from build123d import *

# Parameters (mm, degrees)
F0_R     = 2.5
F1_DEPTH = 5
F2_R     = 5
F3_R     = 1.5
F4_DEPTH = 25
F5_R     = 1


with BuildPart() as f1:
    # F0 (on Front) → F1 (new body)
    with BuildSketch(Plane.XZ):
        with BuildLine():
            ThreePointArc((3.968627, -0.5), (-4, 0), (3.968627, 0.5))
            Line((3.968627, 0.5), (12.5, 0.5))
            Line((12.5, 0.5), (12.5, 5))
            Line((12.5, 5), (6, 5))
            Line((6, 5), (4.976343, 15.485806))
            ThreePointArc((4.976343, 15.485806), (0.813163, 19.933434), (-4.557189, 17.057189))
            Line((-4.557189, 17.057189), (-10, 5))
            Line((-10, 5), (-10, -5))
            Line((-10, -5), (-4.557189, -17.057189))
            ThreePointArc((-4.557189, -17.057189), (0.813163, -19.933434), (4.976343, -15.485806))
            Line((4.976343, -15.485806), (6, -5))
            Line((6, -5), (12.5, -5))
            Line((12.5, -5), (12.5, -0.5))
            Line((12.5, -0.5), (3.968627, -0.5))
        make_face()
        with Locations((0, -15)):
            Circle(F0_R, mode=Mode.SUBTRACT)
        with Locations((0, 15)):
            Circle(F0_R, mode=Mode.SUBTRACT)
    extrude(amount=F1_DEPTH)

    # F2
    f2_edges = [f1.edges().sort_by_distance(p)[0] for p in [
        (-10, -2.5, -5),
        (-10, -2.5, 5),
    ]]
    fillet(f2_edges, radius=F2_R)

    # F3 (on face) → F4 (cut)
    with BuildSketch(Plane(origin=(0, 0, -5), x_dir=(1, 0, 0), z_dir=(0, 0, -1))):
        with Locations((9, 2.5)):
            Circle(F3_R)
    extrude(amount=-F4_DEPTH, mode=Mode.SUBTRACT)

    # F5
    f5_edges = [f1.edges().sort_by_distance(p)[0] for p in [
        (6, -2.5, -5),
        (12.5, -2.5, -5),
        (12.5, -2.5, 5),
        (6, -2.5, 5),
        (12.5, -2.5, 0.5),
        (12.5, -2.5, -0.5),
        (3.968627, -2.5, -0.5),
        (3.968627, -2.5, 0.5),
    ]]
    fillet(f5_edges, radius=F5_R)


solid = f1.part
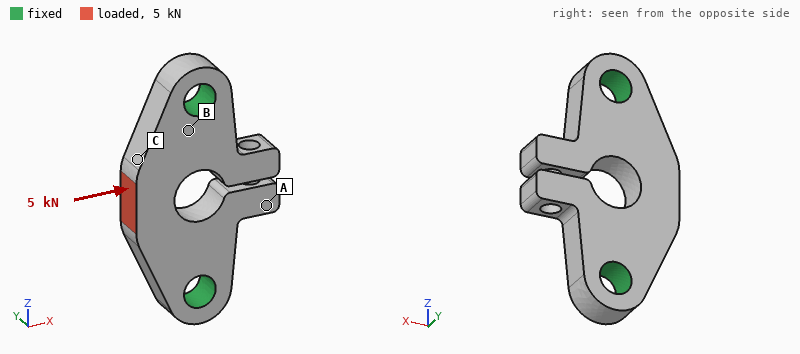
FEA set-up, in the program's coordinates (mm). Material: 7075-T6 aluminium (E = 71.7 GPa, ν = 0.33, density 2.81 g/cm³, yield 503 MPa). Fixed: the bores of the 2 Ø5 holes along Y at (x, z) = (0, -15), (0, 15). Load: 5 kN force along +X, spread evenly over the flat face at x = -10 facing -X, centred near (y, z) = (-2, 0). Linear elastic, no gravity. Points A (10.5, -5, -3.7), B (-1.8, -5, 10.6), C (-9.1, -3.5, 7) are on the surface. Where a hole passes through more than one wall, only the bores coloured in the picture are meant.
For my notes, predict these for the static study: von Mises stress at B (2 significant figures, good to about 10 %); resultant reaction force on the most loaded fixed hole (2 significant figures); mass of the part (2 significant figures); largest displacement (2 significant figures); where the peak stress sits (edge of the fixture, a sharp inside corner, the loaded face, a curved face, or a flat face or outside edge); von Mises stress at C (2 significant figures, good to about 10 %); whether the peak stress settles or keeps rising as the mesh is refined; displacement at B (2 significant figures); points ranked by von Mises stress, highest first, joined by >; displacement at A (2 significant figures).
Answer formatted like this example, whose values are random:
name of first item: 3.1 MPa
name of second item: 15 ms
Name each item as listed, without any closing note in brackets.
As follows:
von Mises stress at B: 110 MPa
resultant reaction force on the most loaded fixed hole: 3.5 kN
mass of the part: 6.4 g
largest displacement: 41 µm
where the peak stress sits: edge of the fixture
von Mises stress at C: 54 MPa
whether the peak stress settles or keeps rising as the mesh is refined: keeps rising
displacement at B: 7.0 µm
points ranked by von Mises stress, highest first, joined by >: B > C > A
displacement at A: 29 µm
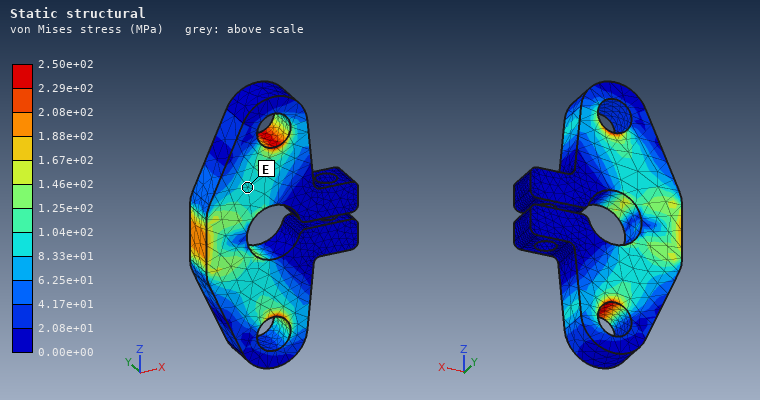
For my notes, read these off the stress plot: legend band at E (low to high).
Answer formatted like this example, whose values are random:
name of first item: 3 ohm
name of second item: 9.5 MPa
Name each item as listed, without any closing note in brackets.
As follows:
legend band at E: 8.33e+01 to 1.04e+02 MPa
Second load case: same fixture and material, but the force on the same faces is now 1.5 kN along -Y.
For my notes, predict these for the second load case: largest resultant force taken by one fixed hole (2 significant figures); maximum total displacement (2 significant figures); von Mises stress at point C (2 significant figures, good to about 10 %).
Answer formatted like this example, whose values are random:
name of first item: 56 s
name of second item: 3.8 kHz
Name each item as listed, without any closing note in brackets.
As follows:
largest resultant force taken by one fixed hole: 750 N
maximum total displacement: 99 µm
von Mises stress at point C: 130 MPa
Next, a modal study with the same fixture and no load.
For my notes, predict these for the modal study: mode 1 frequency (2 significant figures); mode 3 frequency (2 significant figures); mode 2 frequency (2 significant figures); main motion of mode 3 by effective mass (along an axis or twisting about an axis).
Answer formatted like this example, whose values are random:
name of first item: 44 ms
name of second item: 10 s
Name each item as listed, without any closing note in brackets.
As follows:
mode 1 frequency: 17 kHz
mode 3 frequency: 24 kHz
mode 2 frequency: 18 kHz
main motion of mode 3 by effective mass: along Y
